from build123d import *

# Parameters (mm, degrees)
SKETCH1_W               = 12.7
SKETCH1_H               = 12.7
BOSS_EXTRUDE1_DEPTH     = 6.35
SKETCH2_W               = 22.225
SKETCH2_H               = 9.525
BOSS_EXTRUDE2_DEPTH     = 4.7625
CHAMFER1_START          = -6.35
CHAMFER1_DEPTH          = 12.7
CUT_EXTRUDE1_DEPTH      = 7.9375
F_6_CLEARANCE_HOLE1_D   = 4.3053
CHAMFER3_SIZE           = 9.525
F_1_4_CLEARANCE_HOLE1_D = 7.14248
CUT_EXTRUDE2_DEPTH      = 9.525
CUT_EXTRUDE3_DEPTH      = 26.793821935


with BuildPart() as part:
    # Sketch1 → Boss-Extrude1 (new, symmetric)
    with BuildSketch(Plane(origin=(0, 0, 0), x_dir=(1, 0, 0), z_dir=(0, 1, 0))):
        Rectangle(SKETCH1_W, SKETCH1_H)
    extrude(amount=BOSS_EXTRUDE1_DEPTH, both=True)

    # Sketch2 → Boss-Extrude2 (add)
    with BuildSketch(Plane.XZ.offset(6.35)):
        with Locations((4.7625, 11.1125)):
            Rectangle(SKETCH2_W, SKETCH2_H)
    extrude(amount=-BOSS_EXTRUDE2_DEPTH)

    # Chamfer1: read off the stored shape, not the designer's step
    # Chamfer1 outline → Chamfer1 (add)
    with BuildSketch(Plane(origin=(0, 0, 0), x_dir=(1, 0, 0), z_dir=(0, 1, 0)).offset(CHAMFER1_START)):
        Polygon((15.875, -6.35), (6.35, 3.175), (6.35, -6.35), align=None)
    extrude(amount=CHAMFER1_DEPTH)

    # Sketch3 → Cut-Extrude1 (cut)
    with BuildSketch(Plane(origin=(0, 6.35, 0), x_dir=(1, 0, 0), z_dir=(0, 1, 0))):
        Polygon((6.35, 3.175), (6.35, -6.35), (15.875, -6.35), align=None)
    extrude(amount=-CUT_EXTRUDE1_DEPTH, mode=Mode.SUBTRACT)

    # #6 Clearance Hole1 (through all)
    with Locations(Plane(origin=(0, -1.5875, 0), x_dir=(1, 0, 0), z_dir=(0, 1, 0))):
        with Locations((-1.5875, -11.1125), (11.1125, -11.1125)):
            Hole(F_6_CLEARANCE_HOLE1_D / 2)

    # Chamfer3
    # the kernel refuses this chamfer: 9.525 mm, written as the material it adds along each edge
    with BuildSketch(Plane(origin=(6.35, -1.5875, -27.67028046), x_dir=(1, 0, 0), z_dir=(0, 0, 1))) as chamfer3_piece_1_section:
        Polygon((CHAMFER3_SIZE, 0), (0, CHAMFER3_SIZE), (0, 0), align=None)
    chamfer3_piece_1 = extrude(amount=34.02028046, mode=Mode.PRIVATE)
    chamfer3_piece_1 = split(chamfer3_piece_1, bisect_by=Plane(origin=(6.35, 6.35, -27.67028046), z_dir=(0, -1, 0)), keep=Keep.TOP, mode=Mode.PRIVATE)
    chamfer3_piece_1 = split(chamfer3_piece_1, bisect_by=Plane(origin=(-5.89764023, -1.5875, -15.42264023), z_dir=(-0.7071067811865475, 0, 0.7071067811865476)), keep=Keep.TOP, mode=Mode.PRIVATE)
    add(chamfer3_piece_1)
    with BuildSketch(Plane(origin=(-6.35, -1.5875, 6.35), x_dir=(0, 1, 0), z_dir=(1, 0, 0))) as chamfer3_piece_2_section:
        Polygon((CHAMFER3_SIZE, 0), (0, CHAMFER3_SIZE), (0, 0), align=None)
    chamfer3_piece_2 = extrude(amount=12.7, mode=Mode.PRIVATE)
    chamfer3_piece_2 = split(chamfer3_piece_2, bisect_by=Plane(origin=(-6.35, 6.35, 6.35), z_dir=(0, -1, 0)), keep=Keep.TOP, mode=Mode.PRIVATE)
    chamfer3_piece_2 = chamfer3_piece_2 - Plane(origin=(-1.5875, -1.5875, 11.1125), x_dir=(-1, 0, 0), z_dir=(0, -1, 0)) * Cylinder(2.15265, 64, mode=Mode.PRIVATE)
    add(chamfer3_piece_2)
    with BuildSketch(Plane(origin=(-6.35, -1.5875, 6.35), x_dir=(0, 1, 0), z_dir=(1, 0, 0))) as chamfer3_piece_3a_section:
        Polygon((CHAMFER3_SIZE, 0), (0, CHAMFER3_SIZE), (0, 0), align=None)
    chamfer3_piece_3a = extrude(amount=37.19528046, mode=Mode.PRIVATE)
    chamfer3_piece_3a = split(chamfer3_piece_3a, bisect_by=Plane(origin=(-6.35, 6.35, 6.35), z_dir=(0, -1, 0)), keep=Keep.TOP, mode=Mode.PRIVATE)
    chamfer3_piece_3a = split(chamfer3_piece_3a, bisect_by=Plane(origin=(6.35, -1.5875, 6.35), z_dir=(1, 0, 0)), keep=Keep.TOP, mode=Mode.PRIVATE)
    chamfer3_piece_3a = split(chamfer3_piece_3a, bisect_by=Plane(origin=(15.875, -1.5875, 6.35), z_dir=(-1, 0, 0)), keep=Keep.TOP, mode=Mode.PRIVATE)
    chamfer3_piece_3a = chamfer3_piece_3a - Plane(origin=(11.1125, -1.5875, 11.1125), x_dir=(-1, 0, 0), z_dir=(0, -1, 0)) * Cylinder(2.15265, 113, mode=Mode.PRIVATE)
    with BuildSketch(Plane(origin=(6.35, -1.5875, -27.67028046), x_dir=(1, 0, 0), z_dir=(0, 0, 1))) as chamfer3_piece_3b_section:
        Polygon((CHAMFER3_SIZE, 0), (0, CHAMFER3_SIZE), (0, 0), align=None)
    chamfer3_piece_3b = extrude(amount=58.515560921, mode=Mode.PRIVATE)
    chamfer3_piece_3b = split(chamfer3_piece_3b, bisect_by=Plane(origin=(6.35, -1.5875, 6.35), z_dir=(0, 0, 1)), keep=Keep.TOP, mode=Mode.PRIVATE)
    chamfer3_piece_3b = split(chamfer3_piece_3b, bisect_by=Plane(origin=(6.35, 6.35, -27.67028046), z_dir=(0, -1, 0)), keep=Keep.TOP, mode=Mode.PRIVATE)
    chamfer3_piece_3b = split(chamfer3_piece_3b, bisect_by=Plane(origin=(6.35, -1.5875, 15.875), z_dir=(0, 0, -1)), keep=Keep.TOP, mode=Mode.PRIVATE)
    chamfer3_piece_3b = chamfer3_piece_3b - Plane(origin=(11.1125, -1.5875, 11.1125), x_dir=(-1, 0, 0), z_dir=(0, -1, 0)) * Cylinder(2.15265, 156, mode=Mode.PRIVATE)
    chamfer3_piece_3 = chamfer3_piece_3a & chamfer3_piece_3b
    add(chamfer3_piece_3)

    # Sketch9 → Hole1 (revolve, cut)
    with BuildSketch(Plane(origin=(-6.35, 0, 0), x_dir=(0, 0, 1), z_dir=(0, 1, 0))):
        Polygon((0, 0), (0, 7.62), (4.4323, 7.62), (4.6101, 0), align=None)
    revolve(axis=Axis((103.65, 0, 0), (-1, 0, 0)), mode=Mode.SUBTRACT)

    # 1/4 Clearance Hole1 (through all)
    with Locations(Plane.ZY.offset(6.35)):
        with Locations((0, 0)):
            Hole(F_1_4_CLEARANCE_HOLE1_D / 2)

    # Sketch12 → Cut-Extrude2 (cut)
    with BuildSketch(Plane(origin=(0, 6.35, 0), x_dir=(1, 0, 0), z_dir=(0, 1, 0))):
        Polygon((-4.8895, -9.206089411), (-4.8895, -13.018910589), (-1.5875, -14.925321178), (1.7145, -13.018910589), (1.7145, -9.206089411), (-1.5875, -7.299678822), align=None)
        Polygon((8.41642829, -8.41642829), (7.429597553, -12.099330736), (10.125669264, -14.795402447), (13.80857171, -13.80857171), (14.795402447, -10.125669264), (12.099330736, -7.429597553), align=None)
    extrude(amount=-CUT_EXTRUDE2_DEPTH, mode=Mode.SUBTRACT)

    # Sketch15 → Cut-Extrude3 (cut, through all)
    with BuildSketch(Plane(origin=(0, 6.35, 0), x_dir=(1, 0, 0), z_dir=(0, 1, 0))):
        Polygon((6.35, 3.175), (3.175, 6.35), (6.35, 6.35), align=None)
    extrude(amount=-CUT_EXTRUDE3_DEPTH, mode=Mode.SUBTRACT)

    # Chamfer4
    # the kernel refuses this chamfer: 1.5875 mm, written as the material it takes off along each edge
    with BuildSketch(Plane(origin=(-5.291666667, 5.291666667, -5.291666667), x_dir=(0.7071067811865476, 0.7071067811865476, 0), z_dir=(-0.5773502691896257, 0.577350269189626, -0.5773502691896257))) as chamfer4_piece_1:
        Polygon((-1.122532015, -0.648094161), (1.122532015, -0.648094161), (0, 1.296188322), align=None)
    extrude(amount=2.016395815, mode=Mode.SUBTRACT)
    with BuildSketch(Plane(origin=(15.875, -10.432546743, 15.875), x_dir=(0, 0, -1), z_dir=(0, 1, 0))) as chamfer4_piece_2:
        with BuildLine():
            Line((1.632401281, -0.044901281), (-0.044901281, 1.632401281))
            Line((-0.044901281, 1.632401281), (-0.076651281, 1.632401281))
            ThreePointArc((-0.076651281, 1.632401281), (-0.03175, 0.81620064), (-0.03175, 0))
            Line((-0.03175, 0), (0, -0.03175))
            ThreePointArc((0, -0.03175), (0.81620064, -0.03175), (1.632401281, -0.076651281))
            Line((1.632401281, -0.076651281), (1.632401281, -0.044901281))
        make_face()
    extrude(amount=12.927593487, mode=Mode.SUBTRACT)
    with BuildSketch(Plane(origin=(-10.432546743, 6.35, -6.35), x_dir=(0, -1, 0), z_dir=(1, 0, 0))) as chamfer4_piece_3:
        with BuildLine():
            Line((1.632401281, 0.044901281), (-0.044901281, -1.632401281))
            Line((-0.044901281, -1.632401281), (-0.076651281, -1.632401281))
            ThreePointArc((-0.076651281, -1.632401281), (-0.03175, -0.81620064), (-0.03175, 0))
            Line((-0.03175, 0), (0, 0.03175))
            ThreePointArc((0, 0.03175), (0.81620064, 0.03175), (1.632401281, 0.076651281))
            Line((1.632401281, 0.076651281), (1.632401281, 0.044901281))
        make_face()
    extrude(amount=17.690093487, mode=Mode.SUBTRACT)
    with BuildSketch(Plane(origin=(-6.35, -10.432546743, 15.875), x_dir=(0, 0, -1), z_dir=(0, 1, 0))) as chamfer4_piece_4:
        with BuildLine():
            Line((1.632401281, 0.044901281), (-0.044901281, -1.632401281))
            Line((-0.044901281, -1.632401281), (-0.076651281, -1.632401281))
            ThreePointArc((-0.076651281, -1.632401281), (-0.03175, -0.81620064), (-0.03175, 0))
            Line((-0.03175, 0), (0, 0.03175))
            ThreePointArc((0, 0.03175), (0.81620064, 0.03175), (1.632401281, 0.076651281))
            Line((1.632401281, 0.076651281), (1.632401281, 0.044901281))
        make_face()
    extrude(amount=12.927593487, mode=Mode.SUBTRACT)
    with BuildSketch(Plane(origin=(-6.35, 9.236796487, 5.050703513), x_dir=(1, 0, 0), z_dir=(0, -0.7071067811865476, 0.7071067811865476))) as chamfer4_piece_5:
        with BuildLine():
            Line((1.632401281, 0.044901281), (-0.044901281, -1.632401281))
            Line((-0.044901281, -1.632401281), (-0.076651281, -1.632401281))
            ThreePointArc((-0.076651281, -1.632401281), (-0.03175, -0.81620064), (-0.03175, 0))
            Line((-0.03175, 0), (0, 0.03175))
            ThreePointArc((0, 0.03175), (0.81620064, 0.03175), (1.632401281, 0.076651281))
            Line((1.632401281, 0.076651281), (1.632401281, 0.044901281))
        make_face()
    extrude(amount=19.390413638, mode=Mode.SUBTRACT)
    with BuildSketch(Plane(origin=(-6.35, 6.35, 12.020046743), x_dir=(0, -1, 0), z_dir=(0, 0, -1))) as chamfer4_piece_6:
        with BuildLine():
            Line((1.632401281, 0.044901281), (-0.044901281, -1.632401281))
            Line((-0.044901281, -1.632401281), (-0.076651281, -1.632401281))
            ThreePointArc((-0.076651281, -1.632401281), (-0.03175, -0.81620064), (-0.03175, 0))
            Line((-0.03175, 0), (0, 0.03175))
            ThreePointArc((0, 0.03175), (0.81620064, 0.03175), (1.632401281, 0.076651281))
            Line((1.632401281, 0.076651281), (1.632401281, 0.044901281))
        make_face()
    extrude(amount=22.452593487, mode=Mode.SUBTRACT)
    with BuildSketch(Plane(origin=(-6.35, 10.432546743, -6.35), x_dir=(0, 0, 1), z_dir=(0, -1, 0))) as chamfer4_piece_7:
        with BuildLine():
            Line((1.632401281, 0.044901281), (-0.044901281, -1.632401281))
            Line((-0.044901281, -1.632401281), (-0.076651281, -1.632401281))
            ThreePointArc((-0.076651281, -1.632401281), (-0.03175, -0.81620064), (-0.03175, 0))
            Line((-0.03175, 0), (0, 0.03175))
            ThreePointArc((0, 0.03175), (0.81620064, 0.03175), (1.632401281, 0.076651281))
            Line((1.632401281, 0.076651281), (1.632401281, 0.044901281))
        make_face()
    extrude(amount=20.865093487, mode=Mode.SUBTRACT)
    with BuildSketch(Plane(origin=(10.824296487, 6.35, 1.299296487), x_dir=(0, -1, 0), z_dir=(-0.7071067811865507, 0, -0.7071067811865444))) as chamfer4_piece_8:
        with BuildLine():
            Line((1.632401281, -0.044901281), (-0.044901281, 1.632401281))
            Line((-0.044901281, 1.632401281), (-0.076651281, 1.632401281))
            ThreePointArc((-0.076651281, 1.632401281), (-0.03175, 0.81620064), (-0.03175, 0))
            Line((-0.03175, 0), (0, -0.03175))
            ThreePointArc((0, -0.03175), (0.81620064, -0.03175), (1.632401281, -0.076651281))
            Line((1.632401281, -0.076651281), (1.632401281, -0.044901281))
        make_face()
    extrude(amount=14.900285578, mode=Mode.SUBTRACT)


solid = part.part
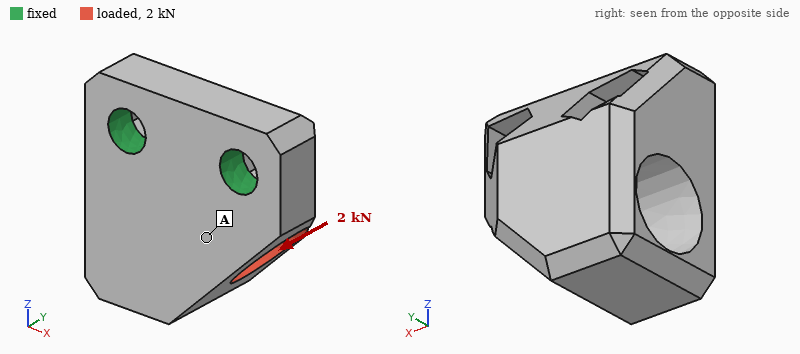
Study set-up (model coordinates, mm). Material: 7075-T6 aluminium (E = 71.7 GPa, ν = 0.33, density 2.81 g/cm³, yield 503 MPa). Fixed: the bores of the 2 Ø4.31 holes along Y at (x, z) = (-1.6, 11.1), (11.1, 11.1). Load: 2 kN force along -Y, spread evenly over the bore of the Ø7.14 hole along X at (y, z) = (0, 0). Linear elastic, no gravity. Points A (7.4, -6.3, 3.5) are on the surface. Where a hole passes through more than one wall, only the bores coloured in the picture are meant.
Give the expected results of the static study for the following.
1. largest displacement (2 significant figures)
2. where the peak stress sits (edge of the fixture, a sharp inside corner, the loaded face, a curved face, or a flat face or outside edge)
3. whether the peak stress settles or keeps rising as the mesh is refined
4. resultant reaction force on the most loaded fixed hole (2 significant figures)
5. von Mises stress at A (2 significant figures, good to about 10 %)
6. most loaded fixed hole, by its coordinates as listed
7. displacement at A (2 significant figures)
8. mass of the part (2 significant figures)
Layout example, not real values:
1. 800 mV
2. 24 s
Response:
1. 0.10 mm
2. edge of the fixture
3. keeps rising
4. 1.2 kN
5. 53 MPa
6. (11.1, 11.1)
7. 0.036 mm
8. 8.2 g
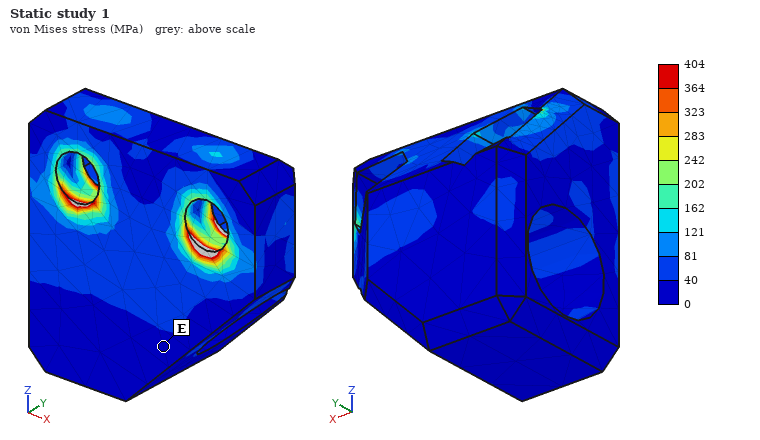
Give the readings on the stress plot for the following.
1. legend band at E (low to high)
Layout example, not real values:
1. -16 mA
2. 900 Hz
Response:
1. 0 to 40 MPa
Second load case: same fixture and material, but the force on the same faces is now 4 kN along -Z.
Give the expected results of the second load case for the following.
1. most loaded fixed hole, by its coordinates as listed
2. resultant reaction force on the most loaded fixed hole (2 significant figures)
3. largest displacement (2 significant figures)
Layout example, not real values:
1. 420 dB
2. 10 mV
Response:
1. (11.1, 11.1)
2. 2.3 kN
3. 90 µm
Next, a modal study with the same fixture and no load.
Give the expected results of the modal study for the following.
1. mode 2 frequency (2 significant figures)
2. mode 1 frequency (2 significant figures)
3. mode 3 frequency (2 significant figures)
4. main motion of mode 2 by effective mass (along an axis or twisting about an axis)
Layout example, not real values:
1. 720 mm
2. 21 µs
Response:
1. 26 kHz
2. 11 kHz
3. 35 kHz
4. along X
